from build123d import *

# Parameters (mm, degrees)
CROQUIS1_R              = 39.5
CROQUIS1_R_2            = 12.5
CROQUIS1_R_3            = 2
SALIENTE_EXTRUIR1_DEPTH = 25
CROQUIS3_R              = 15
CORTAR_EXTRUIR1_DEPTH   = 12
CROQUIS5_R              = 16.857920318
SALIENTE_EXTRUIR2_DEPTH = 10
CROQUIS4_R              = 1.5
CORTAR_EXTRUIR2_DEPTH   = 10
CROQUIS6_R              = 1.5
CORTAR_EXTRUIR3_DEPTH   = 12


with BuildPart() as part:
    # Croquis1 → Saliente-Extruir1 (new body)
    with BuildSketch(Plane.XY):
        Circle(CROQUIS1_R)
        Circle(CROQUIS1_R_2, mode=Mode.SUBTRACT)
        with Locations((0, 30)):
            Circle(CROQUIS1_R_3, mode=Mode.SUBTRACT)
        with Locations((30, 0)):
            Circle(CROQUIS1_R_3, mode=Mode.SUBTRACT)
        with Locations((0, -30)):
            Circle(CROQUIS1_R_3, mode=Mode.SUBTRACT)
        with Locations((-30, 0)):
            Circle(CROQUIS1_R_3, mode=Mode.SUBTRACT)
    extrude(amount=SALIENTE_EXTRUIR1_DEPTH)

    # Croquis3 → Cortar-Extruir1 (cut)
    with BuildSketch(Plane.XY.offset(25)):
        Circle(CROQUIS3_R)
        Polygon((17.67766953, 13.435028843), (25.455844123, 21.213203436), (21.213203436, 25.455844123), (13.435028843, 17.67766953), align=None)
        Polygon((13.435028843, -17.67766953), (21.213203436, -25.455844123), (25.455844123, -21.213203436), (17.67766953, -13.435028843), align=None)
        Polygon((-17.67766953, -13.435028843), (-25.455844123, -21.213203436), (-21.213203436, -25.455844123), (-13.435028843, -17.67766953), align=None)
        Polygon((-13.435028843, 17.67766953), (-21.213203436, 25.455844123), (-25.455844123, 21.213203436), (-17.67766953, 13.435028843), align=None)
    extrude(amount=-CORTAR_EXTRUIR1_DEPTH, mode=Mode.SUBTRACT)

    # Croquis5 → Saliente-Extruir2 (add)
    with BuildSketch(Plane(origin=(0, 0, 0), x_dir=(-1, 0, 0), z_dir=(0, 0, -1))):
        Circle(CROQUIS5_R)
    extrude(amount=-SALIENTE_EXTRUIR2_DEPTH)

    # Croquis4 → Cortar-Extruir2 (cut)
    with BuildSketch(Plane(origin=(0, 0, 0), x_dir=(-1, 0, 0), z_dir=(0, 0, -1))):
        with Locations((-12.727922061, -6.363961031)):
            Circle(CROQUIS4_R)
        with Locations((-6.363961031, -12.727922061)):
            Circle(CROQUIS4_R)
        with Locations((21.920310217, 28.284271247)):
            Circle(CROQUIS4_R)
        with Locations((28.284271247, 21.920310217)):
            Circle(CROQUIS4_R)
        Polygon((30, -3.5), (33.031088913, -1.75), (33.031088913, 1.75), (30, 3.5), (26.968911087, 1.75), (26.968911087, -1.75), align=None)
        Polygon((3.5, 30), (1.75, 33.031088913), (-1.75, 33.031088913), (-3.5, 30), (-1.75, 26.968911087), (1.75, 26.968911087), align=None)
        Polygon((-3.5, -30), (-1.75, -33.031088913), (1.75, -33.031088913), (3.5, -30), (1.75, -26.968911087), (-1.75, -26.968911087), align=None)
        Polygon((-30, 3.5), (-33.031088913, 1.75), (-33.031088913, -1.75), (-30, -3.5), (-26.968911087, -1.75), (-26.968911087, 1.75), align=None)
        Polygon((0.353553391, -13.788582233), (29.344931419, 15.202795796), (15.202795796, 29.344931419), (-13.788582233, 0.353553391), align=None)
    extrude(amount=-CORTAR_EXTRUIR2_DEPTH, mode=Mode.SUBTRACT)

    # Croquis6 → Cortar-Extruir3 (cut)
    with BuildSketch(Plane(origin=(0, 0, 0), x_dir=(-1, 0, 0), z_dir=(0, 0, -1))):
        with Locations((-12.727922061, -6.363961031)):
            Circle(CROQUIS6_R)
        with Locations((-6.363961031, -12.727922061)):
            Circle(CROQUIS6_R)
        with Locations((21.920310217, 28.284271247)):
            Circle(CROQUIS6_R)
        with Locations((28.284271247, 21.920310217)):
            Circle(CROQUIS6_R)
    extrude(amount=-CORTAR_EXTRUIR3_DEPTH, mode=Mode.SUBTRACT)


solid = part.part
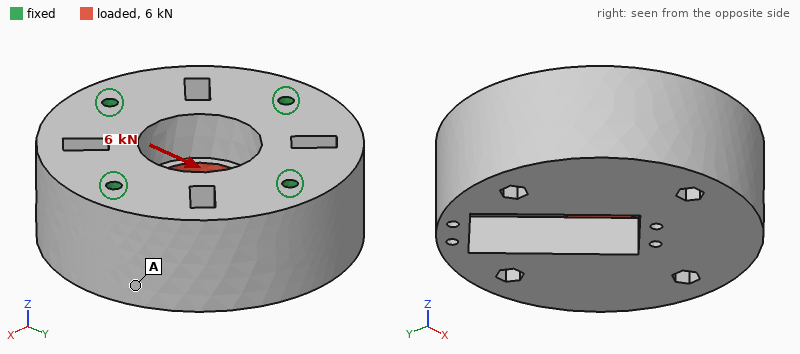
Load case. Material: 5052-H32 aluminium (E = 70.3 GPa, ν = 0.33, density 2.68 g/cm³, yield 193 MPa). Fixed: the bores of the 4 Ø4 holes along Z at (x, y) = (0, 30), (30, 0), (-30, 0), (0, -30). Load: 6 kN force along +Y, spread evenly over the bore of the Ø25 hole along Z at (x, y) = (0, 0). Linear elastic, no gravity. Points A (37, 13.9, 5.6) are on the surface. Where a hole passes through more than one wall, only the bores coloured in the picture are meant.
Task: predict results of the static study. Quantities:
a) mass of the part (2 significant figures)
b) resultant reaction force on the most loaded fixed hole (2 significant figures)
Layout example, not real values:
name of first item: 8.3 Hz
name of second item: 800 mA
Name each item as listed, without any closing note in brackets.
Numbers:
mass of the part: 260 g
resultant reaction force on the most loaded fixed hole: 1.8 kN
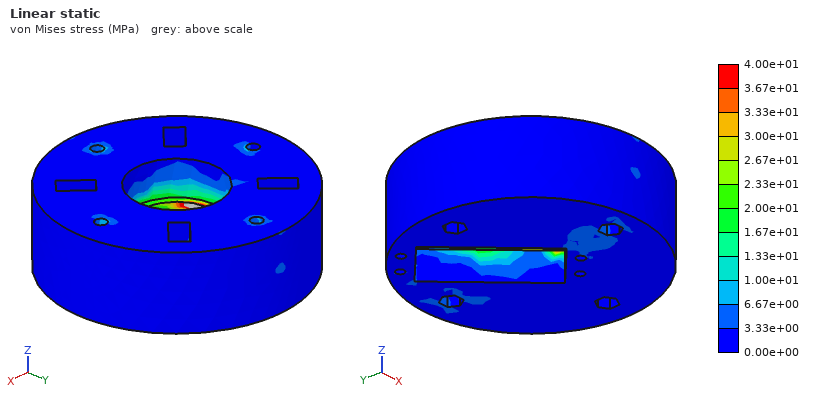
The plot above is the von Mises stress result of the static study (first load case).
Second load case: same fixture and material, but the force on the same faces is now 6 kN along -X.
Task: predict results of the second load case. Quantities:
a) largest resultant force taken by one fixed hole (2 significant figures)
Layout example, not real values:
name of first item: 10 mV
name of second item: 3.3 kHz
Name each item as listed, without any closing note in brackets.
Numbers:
largest resultant force taken by one fixed hole: 1.8 kN
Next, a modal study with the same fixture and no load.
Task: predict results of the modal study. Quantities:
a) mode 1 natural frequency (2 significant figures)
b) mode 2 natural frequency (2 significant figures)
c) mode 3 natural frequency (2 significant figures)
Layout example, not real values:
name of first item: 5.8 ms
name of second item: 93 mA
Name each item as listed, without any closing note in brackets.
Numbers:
mode 1 natural frequency: 16 kHz
mode 2 natural frequency: 18 kHz
mode 3 natural frequency: 19 kHz
